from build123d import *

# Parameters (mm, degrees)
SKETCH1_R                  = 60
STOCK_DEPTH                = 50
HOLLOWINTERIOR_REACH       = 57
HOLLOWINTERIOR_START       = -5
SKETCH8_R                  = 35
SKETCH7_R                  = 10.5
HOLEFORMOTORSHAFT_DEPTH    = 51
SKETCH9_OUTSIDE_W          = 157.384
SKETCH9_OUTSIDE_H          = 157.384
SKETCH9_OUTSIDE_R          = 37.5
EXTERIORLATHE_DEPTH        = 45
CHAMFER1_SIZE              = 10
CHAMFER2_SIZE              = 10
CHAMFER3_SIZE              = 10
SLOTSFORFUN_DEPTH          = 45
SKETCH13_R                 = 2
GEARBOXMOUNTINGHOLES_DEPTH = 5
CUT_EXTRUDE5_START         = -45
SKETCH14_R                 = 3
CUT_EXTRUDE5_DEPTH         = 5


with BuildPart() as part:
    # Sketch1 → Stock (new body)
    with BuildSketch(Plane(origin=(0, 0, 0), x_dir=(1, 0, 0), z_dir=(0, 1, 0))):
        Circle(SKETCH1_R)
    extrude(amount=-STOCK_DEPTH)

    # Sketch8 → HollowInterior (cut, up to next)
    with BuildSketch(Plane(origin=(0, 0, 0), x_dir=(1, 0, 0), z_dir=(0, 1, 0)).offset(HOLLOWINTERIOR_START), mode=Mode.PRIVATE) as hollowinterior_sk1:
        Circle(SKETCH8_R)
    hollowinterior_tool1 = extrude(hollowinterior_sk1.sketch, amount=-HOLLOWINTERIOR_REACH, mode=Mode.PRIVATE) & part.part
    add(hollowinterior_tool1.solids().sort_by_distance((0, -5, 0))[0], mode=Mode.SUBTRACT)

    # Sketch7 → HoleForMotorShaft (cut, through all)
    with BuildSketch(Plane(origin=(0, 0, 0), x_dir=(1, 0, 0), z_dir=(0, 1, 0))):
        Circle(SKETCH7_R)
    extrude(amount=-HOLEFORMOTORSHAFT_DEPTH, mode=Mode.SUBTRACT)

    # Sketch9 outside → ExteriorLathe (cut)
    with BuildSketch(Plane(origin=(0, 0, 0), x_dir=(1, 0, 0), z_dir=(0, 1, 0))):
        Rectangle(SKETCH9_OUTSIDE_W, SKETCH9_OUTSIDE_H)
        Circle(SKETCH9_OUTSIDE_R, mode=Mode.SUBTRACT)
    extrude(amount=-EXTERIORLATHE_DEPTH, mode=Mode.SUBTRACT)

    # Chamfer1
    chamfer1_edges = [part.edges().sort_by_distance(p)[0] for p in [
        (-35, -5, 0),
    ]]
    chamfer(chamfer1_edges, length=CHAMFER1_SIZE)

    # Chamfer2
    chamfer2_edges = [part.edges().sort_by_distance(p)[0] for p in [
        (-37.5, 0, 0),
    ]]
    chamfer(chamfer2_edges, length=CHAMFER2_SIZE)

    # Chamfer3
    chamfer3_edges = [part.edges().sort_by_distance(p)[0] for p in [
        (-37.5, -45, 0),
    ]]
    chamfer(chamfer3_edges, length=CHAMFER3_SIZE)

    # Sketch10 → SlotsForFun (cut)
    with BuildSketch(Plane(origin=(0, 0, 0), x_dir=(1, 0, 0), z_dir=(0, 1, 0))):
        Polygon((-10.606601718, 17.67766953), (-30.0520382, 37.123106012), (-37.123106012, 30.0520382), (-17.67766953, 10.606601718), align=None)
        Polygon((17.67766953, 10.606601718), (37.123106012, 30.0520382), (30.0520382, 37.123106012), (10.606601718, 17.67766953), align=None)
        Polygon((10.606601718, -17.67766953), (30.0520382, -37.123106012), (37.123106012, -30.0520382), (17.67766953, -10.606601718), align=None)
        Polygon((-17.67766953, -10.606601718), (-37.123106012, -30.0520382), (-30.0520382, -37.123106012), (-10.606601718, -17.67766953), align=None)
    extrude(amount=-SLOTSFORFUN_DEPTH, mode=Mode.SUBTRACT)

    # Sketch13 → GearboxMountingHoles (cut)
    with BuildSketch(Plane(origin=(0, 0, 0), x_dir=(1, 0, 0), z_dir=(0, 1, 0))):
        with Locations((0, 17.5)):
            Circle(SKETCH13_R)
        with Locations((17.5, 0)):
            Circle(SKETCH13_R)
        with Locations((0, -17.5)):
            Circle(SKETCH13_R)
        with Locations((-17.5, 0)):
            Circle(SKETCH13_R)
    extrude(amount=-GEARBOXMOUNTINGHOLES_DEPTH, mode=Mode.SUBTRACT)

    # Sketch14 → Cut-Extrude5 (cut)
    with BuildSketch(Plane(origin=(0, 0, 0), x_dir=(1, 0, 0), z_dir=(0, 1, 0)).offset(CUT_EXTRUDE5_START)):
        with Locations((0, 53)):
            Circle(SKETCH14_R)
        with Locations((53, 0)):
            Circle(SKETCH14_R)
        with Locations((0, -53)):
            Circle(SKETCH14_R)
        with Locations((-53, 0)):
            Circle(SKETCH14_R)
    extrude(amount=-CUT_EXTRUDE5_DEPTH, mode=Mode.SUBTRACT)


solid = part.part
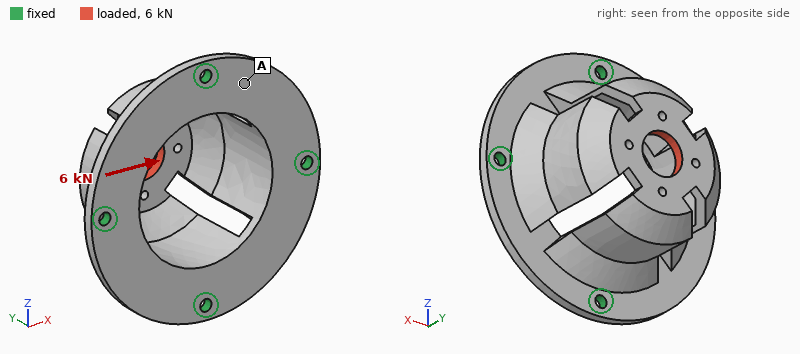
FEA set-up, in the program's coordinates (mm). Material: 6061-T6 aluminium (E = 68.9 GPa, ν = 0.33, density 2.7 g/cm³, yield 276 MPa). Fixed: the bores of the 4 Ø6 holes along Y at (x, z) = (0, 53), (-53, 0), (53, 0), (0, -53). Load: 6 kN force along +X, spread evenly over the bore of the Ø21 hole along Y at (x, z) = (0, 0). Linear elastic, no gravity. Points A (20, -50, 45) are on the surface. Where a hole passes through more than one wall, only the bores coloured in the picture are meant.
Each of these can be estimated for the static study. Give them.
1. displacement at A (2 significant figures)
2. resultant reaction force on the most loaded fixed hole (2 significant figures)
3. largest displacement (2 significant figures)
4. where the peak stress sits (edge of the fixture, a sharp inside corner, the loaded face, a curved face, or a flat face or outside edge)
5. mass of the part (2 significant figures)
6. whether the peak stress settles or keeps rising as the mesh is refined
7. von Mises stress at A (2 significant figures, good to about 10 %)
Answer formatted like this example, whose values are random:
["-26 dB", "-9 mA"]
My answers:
["0.045 mm", "3.2 kN", "0.22 mm", "edge of the fixture", "220 g", "keeps rising", "23 MPa"]
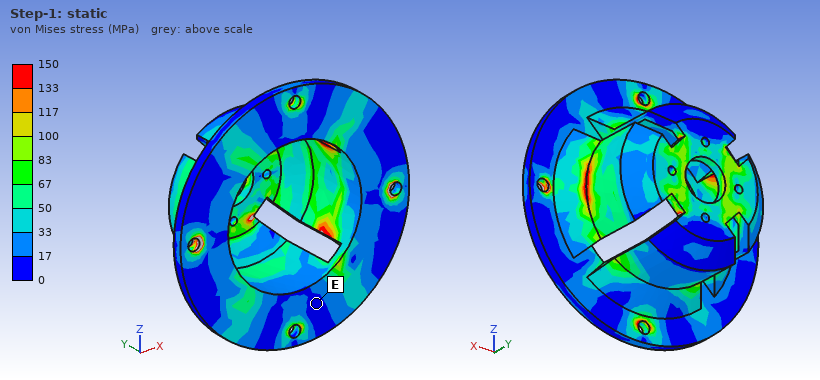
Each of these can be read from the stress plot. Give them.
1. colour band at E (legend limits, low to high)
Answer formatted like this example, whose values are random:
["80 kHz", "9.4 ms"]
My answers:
["0 to 17 MPa"]
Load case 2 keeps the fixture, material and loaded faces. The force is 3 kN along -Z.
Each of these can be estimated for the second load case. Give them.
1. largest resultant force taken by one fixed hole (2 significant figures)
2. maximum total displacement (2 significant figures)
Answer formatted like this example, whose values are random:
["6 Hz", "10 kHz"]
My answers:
["1.6 kN", "0.11 mm"]
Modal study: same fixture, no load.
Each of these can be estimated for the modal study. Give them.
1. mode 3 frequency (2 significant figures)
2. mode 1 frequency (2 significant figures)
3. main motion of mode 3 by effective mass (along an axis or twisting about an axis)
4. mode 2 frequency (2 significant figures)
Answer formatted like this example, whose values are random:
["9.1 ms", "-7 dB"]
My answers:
["4600 Hz", "3500 Hz", "along Y", "3600 Hz"]
